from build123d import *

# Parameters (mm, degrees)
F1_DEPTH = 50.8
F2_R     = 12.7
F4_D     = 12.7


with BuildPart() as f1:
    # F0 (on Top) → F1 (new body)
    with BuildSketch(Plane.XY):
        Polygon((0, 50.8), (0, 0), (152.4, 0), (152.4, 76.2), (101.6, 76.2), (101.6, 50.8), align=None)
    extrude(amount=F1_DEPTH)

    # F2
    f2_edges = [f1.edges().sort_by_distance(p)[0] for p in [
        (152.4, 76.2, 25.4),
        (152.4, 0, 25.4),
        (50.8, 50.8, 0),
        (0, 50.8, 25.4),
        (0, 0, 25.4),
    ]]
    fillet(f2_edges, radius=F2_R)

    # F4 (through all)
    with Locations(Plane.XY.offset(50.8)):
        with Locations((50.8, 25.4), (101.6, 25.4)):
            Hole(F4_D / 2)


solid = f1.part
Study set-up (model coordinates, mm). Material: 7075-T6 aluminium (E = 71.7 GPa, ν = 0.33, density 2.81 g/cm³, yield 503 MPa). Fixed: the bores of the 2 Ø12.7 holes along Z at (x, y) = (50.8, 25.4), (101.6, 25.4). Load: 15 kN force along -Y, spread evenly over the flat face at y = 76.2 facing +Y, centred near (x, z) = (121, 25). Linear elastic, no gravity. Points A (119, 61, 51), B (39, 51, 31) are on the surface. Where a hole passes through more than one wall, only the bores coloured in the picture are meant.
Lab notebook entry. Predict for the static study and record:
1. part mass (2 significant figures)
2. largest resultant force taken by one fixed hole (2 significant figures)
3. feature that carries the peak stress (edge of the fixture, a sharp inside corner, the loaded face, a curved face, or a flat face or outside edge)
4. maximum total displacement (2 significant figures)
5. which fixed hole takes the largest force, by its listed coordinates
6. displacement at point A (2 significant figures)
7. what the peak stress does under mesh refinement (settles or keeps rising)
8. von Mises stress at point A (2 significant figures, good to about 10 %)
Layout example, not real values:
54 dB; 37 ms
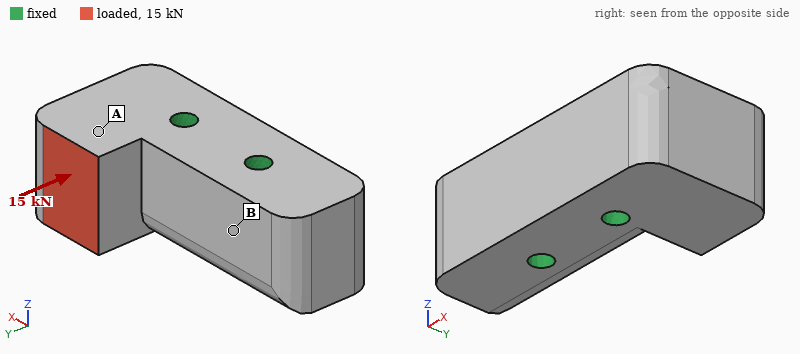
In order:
1.2 kg; 18 kN; edge of the fixture; 20 µm; (101.6, 25.4); 13 µm; keeps rising; 8.1 MPa
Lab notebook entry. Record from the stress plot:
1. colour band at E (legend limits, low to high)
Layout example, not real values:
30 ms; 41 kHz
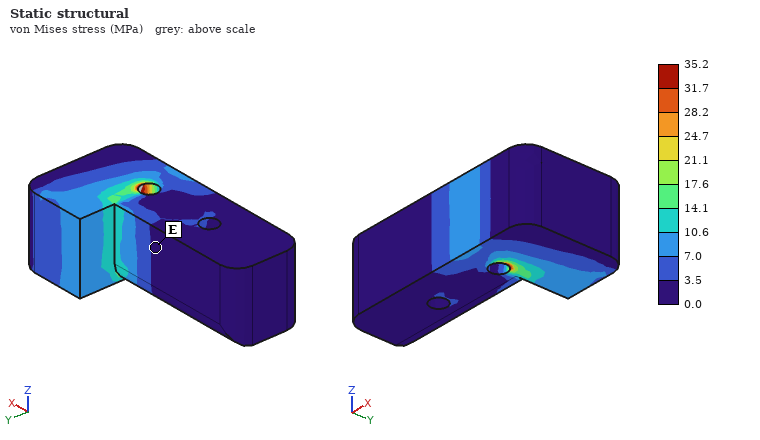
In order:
0.0 to 3.5 MPa
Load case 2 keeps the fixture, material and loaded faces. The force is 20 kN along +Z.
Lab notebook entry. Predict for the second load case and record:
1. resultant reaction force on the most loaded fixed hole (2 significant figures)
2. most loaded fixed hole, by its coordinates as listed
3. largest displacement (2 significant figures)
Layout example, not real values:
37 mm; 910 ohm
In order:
20 kN; (101.6, 25.4); 67 µm
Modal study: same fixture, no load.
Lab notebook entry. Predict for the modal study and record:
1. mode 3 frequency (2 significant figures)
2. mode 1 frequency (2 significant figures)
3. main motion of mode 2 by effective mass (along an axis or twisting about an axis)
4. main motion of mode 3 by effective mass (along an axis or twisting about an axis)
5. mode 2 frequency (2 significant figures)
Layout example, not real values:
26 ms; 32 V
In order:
8200 Hz; 5700 Hz; along Z; along Y; 7300 Hz
